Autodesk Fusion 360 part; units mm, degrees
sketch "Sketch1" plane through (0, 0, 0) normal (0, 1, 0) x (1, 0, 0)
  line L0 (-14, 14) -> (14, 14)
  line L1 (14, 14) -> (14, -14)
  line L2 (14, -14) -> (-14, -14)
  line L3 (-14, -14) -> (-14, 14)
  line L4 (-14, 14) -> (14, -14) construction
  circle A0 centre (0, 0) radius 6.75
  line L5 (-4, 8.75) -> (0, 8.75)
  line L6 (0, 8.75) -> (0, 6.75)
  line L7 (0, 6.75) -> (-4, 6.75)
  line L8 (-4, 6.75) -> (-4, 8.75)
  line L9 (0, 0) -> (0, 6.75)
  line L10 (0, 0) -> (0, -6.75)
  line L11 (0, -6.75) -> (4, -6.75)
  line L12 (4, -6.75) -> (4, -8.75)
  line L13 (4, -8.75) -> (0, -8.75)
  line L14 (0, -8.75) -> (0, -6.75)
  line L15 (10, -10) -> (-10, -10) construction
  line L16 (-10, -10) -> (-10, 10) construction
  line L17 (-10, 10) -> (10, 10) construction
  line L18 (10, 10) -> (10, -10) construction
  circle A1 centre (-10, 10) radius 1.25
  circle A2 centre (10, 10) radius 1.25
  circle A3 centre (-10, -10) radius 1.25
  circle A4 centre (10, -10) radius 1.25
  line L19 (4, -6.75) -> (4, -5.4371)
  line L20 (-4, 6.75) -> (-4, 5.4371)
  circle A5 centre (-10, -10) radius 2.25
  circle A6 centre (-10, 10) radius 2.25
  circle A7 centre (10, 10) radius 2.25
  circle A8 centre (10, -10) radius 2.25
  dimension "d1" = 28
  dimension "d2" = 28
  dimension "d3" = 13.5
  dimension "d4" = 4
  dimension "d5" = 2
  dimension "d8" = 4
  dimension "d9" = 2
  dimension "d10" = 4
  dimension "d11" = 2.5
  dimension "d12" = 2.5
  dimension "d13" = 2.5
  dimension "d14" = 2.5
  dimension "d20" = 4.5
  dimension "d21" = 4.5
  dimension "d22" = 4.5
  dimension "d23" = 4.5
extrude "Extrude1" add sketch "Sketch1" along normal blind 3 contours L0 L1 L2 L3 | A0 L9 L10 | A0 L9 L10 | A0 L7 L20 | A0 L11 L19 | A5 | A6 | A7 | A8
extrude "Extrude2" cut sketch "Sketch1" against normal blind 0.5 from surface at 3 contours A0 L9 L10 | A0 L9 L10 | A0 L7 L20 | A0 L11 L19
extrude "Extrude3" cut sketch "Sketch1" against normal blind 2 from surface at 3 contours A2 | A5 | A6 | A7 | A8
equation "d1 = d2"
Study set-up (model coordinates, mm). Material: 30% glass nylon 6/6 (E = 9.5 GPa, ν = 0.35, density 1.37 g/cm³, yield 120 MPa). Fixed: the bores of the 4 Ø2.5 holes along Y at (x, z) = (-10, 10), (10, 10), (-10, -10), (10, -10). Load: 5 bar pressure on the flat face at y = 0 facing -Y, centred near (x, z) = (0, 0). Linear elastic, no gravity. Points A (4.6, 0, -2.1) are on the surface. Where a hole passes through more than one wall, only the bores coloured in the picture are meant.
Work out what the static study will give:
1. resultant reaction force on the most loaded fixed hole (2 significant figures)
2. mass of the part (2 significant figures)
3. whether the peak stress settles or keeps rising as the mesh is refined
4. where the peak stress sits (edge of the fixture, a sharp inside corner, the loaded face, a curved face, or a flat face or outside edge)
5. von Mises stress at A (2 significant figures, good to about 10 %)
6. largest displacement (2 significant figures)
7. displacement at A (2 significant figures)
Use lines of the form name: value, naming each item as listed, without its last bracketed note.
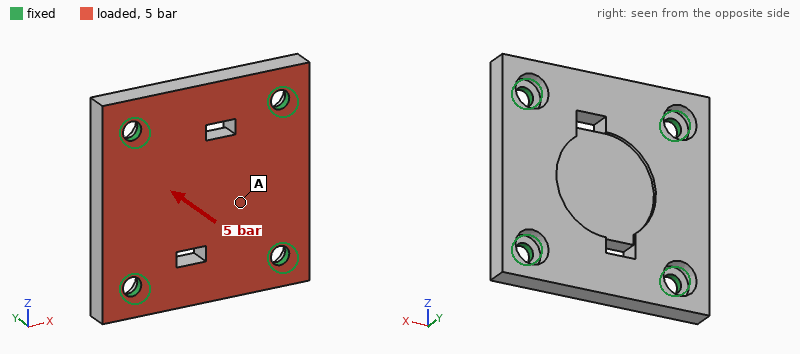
resultant reaction force on the most loaded fixed hole: 110 N
mass of the part: 2.9 g
whether the peak stress settles or keeps rising as the mesh is refined: keeps rising
where the peak stress sits: edge of the fixture
von Mises stress at A: 6.8 MPa
largest displacement: 47 µm
displacement at A: 40 µm
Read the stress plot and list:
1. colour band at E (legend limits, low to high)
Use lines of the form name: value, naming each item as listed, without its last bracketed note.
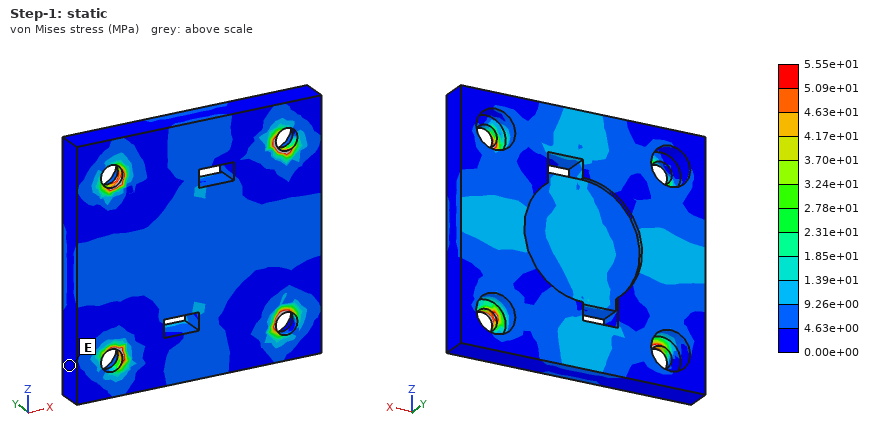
colour band at E: 0.00e+00 to 4.63e+00 MPa
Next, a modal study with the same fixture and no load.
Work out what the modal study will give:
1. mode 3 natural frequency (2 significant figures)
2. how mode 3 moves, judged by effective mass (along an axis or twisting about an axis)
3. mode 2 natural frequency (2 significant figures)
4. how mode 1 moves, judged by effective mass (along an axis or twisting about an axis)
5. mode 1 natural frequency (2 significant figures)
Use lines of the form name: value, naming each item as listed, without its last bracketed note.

mode 3 natural frequency: 15 kHz
how mode 3 moves, judged by effective mass: twisting about Z
mode 2 natural frequency: 14 kHz
how mode 1 moves, judged by effective mass: along Y
mode 1 natural frequency: 10 kHz
